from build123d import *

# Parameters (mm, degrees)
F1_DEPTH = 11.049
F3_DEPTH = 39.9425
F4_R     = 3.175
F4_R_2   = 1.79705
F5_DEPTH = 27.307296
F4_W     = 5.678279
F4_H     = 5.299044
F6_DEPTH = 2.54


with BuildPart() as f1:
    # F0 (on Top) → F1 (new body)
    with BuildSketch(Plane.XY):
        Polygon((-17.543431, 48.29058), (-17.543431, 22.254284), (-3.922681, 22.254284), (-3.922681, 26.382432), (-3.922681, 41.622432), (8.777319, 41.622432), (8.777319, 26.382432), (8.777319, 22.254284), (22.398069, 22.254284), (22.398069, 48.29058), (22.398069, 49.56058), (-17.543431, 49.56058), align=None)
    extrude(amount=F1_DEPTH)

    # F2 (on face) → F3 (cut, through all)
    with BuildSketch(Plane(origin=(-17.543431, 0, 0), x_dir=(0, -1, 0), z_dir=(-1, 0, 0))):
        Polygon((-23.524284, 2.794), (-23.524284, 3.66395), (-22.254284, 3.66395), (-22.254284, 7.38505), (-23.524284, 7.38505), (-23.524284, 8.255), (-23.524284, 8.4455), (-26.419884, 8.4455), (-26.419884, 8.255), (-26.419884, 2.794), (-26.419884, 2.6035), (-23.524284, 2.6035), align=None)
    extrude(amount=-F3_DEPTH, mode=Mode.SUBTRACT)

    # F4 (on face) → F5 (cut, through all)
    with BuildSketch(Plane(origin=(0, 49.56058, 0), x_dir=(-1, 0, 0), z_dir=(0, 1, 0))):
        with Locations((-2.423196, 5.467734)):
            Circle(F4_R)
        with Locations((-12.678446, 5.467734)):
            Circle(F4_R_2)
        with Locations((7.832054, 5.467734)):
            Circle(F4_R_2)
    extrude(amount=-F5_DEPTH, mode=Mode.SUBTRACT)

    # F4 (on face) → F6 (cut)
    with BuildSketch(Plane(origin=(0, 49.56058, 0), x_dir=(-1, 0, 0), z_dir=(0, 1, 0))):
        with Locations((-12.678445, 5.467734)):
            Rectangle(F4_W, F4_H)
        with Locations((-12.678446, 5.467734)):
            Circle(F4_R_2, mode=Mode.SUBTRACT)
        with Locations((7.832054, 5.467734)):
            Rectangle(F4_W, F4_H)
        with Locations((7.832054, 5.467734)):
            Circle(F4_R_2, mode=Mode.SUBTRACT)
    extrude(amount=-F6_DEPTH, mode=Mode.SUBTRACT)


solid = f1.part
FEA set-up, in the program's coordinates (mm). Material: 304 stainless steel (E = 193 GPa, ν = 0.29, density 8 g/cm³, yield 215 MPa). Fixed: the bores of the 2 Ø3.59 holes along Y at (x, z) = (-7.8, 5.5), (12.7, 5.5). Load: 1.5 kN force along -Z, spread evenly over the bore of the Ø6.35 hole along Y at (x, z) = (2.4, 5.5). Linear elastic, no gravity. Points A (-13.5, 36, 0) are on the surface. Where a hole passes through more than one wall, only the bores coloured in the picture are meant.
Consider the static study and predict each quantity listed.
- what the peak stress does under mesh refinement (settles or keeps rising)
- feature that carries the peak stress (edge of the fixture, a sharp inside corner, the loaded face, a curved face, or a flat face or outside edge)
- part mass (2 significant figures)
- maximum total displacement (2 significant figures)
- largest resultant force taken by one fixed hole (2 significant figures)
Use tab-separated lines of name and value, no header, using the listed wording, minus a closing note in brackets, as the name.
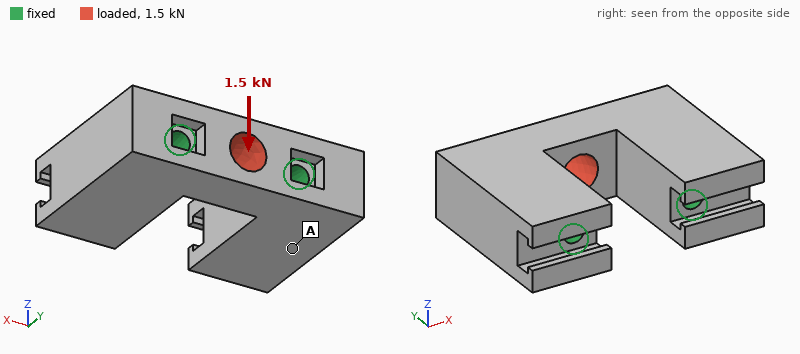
what the peak stress does under mesh refinement	keeps rising
feature that carries the peak stress	edge of the fixture
part mass	63 g
maximum total displacement	2.3 µm
largest resultant force taken by one fixed hole	750 N
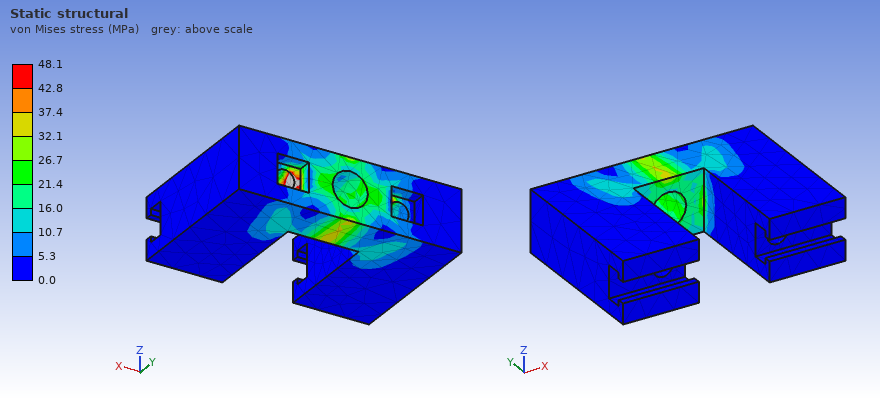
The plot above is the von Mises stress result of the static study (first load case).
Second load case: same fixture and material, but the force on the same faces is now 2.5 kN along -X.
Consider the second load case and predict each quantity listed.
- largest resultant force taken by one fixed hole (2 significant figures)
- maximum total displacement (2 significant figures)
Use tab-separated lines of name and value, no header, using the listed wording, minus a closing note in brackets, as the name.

largest resultant force taken by one fixed hole	1.3 kN
maximum total displacement	0.98 µm
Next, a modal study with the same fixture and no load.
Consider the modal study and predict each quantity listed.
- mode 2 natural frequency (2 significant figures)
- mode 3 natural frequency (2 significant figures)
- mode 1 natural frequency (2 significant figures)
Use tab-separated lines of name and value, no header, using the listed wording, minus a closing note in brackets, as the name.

mode 2 natural frequency	37 kHz
mode 3 natural frequency	46 kHz
mode 1 natural frequency	37 kHz
